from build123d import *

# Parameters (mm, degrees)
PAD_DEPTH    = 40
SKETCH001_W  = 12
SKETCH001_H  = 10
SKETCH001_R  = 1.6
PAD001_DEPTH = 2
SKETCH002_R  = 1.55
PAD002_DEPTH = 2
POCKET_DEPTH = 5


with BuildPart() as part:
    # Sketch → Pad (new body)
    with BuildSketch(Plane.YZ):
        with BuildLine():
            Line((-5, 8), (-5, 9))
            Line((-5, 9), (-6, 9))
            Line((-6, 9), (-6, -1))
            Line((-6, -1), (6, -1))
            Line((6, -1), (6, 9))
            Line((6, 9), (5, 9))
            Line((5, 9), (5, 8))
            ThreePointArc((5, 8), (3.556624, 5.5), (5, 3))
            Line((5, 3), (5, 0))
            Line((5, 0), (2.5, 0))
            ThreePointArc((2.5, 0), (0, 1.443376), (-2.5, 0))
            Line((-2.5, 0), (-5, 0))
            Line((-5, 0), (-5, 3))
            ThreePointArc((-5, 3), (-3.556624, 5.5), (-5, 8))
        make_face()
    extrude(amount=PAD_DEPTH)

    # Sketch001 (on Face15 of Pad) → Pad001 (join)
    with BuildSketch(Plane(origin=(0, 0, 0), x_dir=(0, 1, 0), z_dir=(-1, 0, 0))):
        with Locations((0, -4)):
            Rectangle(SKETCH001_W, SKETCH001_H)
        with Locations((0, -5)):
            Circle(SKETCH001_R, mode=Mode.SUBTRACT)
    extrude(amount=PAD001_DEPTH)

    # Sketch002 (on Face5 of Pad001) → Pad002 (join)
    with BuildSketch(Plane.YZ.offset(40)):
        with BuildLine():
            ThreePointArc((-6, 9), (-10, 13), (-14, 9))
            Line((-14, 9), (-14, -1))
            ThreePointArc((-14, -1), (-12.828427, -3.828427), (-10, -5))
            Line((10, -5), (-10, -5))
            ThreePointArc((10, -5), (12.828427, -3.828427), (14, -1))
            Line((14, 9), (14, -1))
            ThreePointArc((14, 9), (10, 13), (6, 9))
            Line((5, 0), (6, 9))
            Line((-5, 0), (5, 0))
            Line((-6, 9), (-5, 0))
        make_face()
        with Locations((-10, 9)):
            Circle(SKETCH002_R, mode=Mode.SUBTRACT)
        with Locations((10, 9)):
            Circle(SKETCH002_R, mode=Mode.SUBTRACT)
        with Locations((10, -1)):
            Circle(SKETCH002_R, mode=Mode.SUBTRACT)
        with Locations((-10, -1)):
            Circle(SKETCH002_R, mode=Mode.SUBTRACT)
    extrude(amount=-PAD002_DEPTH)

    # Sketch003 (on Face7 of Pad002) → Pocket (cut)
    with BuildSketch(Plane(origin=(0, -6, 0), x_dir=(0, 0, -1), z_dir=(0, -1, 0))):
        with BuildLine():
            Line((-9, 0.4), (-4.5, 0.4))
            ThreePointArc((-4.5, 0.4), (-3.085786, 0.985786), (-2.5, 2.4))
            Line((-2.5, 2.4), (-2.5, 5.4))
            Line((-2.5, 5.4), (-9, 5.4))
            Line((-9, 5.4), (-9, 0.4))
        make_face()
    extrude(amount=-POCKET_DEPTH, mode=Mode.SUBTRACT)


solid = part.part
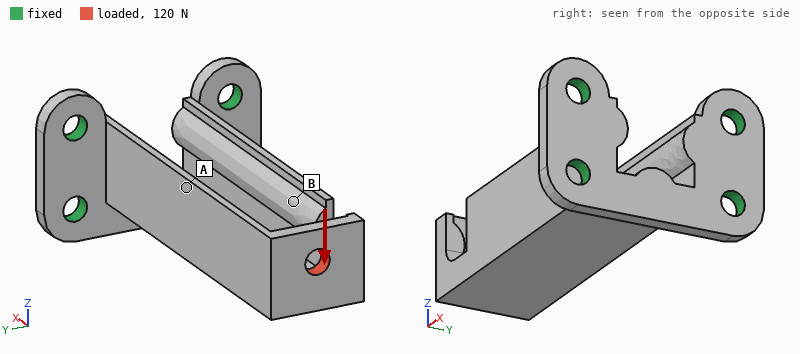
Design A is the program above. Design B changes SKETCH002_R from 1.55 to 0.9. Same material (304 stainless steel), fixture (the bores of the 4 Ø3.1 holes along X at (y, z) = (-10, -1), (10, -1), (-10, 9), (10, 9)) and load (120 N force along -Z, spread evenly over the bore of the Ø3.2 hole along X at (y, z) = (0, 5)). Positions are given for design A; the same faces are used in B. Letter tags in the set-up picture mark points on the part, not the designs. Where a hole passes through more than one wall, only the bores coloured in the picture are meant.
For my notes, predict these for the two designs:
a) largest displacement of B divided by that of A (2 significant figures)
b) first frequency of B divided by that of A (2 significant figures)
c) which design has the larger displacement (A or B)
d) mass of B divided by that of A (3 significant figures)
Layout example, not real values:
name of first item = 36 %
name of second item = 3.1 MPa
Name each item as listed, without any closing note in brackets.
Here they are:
largest displacement of B divided by that of A = 1.2
first frequency of B divided by that of A = 0.95
which design has the larger displacement = B
mass of B divided by that of A = 1.02
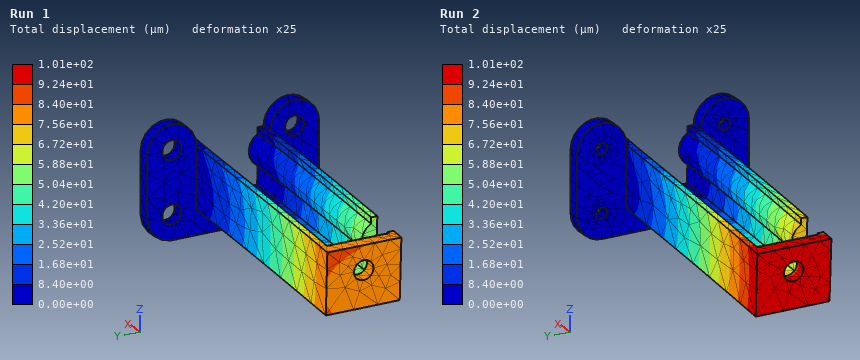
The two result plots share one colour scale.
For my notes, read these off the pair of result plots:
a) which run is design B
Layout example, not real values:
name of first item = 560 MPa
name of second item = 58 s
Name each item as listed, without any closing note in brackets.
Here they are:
which run is design B = Run 2
